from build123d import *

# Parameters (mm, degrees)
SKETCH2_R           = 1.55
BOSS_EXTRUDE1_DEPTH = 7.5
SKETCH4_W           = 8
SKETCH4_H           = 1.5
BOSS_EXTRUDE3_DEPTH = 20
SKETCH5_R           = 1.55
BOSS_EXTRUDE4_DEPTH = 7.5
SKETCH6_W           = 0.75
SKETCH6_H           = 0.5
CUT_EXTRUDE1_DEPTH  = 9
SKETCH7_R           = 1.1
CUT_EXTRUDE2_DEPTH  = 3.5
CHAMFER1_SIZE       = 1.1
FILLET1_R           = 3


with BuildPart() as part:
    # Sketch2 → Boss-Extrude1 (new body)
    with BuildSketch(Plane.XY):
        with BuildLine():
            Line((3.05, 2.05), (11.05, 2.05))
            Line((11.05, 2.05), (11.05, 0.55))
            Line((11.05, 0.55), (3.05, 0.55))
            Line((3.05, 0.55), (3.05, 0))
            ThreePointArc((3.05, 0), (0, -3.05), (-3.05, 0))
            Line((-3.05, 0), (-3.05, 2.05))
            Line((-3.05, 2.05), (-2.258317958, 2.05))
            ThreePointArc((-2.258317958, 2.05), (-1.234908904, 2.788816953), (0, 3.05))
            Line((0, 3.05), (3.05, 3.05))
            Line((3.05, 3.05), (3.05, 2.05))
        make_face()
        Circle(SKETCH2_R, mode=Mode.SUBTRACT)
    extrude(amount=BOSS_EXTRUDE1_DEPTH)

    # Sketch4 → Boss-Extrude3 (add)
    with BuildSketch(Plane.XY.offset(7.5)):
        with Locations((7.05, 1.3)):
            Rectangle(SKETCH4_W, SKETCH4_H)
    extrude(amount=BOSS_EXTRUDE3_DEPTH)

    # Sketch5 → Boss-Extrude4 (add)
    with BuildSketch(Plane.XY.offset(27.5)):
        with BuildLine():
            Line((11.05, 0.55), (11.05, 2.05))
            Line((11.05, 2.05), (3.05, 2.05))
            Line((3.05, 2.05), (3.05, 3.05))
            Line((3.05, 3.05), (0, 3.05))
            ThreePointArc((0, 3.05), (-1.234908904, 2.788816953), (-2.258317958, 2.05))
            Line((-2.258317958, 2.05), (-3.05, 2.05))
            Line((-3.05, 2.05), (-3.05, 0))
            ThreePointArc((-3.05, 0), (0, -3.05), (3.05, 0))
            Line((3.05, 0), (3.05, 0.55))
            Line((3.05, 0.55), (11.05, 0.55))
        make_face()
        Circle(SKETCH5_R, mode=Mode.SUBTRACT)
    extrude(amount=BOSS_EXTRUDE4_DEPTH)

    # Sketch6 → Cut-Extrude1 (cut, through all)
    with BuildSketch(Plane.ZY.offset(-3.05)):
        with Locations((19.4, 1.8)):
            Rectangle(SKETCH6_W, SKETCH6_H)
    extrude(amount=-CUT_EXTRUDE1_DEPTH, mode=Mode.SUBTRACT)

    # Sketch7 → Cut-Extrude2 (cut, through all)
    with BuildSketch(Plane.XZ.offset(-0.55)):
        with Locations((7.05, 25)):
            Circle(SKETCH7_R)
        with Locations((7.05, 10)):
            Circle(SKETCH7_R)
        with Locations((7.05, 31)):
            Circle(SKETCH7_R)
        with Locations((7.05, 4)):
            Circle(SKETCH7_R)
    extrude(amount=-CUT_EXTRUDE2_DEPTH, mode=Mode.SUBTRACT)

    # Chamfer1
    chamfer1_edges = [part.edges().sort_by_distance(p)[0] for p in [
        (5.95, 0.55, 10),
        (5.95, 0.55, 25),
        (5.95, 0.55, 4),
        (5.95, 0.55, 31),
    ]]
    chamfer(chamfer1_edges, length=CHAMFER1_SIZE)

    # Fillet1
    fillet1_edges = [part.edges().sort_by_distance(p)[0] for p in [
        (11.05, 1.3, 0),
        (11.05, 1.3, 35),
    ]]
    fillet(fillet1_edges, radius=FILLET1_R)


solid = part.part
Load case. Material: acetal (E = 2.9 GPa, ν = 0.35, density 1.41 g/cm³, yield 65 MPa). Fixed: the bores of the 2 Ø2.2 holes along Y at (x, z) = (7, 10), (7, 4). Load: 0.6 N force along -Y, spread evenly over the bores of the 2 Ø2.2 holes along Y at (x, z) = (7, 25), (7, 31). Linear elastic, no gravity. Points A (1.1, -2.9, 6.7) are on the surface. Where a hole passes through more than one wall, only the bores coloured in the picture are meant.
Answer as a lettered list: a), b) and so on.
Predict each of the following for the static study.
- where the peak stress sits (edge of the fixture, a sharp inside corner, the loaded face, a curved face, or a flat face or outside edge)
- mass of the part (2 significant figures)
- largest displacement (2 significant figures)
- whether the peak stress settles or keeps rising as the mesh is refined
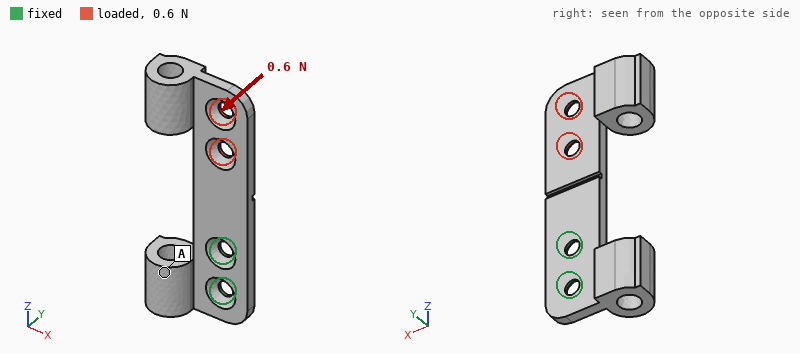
a) edge of the fixture
b) 1.0 g
c) 0.39 mm
d) keeps rising
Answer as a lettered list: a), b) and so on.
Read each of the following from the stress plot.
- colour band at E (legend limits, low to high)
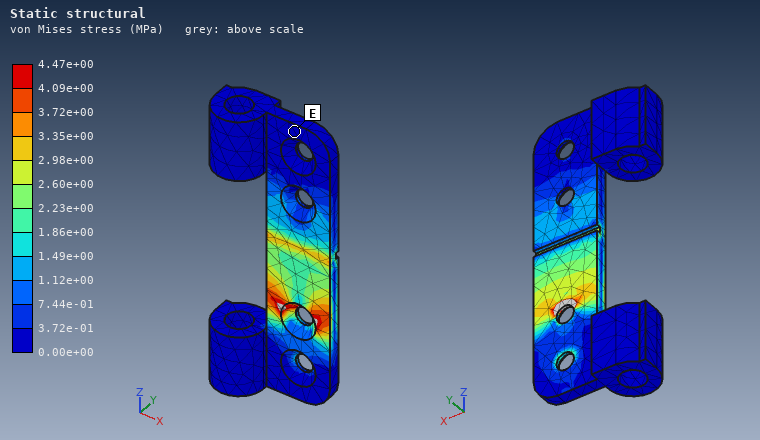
a) 0.00e+00 to 3.72e-01 MPa
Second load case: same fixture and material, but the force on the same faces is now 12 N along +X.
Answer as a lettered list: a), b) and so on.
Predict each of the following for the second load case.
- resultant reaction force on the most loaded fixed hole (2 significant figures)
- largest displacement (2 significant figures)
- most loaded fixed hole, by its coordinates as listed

a) 36 N
b) 0.43 mm
c) (7, 10)
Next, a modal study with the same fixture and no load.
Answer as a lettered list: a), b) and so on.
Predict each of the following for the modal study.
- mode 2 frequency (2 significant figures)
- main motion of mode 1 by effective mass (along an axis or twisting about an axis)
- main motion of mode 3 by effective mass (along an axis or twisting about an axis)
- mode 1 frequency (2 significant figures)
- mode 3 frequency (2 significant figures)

a) 1100 Hz
b) along Y
c) along X
d) 290 Hz
e) 1400 Hz
